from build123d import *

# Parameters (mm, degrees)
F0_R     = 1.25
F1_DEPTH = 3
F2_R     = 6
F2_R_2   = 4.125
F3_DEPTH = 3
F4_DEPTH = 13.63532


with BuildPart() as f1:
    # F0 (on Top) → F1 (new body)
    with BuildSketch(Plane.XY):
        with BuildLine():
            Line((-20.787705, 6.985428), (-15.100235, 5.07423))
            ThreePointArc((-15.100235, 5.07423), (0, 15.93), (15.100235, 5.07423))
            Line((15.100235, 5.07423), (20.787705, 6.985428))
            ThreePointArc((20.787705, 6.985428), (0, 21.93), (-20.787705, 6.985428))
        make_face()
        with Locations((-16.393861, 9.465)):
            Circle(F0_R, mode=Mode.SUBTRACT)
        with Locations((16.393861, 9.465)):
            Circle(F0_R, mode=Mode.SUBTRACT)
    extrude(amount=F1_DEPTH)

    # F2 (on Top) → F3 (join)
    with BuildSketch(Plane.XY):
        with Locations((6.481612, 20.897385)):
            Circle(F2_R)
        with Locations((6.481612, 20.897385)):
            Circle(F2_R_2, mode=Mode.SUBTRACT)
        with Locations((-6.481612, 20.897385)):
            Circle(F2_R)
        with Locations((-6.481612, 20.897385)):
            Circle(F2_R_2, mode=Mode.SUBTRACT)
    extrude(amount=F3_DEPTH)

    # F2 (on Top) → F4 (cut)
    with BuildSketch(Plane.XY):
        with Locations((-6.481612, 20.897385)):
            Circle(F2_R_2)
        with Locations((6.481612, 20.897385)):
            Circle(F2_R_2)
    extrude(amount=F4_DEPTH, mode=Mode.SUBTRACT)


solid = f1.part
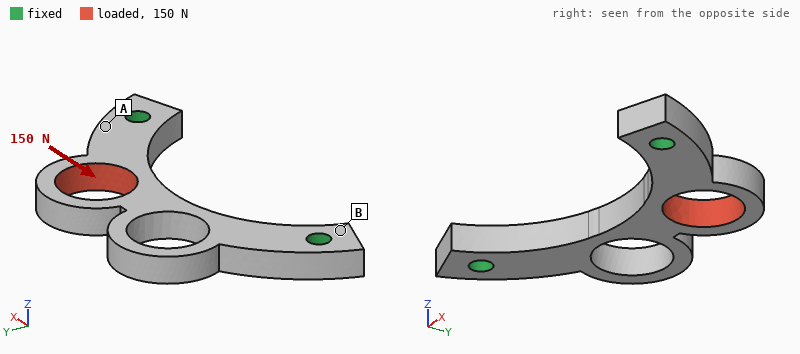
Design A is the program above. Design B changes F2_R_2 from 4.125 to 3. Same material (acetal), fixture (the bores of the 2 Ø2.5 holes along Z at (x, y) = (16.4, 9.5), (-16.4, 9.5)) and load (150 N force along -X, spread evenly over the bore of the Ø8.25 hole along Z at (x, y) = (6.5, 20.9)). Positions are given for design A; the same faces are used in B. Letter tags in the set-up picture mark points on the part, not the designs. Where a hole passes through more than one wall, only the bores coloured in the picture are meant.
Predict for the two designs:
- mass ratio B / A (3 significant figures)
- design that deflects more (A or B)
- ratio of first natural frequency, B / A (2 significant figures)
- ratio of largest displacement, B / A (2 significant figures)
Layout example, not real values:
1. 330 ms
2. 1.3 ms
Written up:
1. 1.18
2. A
3. 0.93
4. 0.44
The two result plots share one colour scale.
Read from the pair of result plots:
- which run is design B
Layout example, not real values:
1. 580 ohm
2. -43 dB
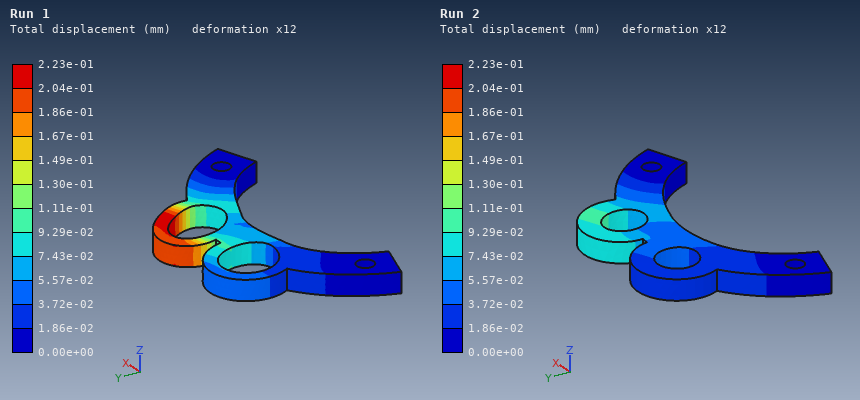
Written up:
1. Run 2
